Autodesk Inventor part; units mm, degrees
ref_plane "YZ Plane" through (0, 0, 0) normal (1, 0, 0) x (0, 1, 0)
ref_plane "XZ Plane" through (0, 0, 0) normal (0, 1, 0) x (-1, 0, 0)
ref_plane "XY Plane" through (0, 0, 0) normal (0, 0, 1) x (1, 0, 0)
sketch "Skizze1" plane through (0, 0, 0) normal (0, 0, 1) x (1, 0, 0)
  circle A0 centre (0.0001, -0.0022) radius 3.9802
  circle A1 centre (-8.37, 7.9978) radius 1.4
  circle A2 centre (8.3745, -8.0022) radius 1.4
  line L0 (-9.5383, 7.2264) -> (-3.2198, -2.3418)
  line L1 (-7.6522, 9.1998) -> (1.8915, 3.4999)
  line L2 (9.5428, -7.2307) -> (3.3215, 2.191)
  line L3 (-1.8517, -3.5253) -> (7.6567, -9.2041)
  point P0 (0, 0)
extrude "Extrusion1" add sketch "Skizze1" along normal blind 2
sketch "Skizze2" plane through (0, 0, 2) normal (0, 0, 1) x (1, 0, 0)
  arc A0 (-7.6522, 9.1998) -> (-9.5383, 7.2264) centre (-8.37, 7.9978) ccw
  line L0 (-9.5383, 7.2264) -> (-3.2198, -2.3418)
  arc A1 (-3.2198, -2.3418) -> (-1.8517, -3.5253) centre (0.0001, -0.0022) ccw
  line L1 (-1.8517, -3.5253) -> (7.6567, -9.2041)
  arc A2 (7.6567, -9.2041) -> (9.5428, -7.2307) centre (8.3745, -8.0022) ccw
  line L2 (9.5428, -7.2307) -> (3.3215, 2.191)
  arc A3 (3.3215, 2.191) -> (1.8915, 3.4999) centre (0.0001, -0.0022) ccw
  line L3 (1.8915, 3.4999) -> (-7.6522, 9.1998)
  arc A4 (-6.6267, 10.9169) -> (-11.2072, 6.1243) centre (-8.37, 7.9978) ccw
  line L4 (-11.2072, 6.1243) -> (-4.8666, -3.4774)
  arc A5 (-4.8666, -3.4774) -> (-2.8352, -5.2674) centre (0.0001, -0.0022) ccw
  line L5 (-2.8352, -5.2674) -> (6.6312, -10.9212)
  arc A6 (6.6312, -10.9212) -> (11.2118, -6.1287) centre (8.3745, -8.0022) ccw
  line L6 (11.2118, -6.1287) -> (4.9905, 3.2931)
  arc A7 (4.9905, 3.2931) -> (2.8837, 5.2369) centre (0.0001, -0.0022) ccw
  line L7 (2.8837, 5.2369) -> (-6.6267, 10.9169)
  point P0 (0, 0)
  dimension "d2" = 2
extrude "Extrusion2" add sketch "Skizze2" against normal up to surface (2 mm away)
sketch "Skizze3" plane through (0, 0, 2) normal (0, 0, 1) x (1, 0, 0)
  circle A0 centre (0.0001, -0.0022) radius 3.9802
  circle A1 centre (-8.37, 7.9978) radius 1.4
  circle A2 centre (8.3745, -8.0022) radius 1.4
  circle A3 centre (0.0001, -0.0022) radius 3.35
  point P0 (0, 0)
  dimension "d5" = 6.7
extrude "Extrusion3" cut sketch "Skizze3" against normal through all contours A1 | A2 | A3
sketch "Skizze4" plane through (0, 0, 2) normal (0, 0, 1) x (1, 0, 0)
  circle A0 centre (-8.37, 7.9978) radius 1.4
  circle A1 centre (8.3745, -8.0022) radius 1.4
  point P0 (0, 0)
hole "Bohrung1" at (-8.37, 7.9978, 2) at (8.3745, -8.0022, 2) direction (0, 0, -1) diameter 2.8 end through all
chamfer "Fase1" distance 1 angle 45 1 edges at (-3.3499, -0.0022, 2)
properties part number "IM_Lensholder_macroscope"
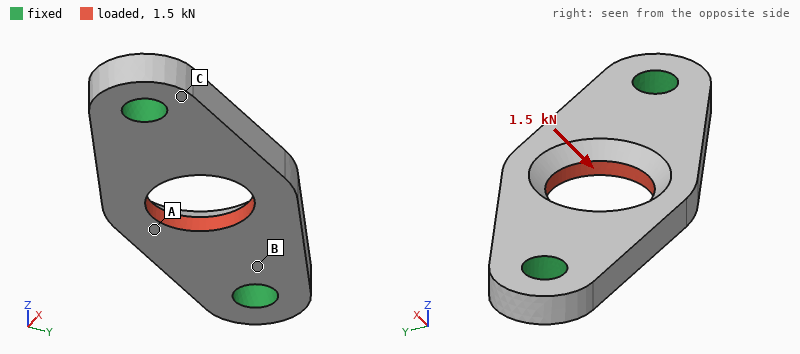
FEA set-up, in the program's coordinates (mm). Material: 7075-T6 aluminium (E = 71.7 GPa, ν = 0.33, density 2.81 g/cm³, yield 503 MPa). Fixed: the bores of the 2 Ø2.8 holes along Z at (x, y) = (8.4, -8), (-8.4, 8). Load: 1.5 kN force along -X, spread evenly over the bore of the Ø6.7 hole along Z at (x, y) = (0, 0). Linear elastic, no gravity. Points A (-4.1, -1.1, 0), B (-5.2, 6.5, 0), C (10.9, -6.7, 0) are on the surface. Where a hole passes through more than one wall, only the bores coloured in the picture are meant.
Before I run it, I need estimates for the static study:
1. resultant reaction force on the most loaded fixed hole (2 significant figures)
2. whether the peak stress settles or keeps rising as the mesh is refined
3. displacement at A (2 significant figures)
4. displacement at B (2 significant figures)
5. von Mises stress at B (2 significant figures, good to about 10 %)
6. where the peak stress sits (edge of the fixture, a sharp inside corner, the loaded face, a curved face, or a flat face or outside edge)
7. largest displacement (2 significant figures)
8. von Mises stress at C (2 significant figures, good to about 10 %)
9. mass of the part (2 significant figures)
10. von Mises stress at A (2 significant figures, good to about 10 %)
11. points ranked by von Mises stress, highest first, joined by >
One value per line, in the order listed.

750 N
keeps rising
27 µm
7.2 µm
120 MPa
edge of the fixture
32 µm
29 MPa
1.2 g
90 MPa
B > A > C
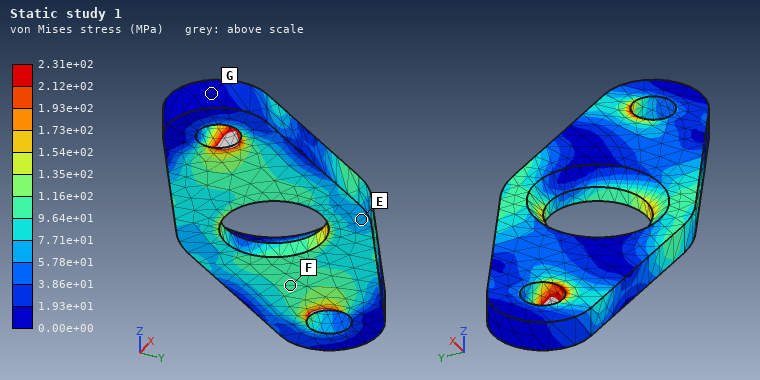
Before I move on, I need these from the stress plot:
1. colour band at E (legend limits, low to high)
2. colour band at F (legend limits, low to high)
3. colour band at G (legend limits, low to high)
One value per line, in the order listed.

5.78e+01 to 7.71e+01 MPa
9.64e+01 to 1.16e+02 MPa
0.00e+00 to 1.93e+01 MPa
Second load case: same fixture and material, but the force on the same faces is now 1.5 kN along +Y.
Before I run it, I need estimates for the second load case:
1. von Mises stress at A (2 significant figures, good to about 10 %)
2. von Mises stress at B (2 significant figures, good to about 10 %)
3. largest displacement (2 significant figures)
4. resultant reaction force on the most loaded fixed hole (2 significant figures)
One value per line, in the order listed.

85 MPa
110 MPa
34 µm
750 N
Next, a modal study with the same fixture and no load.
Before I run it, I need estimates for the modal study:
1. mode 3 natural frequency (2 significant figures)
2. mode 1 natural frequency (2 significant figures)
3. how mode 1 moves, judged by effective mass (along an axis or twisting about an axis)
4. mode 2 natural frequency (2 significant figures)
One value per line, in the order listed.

46 kHz
20 kHz
along Z
24 kHz
